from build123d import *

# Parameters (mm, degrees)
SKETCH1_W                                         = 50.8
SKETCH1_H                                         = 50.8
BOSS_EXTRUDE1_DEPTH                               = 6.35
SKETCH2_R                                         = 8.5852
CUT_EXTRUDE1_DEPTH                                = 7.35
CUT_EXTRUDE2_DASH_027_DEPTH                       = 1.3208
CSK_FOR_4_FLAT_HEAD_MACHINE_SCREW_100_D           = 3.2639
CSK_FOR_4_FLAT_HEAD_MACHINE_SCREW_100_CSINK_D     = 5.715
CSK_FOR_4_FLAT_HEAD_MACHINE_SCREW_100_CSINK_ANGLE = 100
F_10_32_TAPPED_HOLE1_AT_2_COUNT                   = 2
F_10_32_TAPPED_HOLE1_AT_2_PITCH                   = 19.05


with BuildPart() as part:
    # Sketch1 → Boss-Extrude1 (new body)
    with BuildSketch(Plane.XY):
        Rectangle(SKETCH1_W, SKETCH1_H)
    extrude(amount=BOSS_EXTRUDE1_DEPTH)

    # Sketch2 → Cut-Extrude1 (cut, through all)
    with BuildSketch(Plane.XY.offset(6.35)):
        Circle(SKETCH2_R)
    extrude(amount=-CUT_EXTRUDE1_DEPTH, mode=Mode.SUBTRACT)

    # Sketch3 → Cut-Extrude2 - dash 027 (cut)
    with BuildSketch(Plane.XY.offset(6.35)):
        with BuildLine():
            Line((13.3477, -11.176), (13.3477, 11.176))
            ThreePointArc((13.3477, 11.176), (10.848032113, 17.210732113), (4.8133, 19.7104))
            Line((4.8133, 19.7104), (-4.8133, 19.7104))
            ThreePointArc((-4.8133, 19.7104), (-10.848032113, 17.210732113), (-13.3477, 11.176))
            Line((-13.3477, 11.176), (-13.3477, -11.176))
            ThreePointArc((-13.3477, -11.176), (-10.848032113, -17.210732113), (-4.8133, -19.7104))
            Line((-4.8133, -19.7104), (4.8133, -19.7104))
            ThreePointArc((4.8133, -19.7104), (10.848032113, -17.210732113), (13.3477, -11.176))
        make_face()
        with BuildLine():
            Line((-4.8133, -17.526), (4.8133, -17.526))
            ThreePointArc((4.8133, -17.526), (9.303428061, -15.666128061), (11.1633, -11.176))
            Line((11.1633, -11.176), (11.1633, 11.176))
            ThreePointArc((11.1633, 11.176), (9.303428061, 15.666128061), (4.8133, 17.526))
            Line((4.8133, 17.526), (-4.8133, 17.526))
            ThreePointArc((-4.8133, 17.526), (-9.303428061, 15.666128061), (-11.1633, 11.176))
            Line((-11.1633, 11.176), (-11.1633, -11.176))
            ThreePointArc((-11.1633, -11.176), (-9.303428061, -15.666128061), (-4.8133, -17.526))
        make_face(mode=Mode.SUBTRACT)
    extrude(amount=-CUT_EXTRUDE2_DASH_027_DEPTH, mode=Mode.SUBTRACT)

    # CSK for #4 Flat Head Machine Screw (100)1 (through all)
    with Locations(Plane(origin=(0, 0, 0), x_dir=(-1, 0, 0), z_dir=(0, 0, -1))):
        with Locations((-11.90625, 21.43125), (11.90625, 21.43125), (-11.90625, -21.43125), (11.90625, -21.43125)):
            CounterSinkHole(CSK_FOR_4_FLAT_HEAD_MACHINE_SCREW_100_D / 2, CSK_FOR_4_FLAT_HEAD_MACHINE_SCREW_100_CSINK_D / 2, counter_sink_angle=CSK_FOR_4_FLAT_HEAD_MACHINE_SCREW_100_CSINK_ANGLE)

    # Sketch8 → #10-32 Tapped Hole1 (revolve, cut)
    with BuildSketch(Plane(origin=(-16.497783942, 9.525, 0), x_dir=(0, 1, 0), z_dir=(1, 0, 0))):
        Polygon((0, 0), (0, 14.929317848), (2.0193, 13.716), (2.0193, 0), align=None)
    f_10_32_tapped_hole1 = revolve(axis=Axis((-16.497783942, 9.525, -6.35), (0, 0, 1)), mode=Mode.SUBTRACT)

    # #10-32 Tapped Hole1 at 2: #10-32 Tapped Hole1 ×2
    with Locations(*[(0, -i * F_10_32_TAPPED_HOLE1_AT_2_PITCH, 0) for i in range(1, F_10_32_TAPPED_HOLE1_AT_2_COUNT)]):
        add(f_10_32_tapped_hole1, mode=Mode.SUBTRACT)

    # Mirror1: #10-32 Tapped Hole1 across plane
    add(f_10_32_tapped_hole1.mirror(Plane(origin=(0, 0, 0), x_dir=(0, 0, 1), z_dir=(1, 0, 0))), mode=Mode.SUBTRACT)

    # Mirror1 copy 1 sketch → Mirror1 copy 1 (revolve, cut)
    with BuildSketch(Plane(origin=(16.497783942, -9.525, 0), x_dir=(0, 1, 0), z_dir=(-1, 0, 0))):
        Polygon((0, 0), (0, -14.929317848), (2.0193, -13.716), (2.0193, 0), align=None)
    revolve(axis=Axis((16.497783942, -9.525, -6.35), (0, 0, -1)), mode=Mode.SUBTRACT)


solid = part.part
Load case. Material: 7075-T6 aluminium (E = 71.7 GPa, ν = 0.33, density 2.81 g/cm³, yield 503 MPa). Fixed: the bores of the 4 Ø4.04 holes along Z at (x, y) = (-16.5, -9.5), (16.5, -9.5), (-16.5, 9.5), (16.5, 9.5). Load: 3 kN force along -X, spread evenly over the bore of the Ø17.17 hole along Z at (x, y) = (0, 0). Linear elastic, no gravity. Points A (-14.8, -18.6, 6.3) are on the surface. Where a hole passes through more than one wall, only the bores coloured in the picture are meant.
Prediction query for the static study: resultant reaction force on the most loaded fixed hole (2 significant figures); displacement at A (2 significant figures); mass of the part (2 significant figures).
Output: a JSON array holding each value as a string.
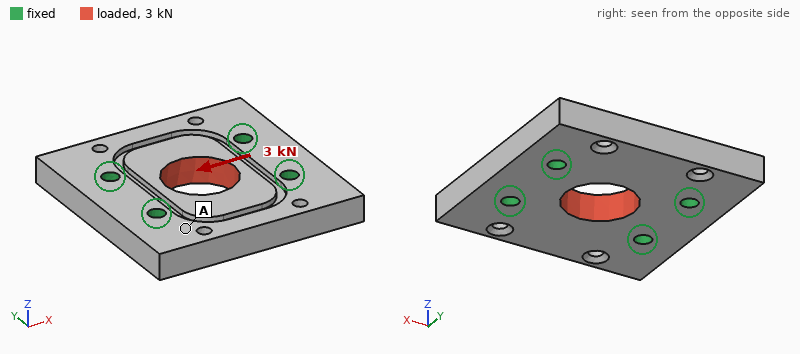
["770 N", "0.58 µm", "39 g"]
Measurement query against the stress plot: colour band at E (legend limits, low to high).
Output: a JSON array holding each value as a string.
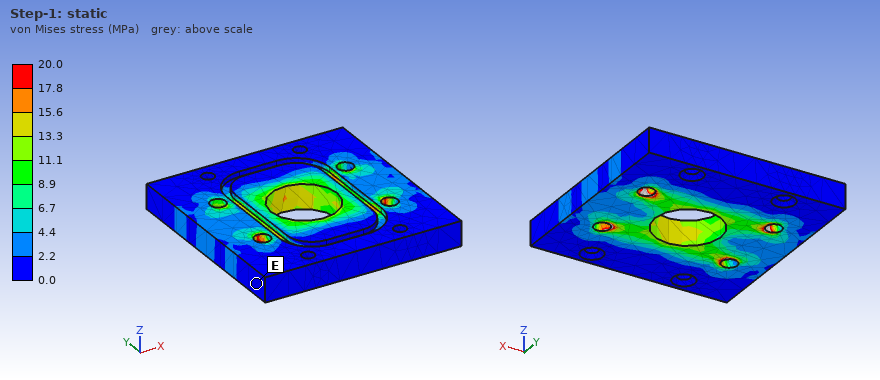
["0.0 to 2.2 MPa"]
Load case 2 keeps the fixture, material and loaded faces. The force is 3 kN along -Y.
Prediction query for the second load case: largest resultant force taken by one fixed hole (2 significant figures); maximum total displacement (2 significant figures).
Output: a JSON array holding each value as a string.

["760 N", "3.8 µm"]
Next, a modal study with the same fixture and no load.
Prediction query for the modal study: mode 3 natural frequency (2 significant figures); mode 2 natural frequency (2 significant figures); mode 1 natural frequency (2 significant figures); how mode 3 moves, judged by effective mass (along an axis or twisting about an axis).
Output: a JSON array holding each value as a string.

["21 kHz", "15 kHz", "14 kHz", "twisting about Y"]
